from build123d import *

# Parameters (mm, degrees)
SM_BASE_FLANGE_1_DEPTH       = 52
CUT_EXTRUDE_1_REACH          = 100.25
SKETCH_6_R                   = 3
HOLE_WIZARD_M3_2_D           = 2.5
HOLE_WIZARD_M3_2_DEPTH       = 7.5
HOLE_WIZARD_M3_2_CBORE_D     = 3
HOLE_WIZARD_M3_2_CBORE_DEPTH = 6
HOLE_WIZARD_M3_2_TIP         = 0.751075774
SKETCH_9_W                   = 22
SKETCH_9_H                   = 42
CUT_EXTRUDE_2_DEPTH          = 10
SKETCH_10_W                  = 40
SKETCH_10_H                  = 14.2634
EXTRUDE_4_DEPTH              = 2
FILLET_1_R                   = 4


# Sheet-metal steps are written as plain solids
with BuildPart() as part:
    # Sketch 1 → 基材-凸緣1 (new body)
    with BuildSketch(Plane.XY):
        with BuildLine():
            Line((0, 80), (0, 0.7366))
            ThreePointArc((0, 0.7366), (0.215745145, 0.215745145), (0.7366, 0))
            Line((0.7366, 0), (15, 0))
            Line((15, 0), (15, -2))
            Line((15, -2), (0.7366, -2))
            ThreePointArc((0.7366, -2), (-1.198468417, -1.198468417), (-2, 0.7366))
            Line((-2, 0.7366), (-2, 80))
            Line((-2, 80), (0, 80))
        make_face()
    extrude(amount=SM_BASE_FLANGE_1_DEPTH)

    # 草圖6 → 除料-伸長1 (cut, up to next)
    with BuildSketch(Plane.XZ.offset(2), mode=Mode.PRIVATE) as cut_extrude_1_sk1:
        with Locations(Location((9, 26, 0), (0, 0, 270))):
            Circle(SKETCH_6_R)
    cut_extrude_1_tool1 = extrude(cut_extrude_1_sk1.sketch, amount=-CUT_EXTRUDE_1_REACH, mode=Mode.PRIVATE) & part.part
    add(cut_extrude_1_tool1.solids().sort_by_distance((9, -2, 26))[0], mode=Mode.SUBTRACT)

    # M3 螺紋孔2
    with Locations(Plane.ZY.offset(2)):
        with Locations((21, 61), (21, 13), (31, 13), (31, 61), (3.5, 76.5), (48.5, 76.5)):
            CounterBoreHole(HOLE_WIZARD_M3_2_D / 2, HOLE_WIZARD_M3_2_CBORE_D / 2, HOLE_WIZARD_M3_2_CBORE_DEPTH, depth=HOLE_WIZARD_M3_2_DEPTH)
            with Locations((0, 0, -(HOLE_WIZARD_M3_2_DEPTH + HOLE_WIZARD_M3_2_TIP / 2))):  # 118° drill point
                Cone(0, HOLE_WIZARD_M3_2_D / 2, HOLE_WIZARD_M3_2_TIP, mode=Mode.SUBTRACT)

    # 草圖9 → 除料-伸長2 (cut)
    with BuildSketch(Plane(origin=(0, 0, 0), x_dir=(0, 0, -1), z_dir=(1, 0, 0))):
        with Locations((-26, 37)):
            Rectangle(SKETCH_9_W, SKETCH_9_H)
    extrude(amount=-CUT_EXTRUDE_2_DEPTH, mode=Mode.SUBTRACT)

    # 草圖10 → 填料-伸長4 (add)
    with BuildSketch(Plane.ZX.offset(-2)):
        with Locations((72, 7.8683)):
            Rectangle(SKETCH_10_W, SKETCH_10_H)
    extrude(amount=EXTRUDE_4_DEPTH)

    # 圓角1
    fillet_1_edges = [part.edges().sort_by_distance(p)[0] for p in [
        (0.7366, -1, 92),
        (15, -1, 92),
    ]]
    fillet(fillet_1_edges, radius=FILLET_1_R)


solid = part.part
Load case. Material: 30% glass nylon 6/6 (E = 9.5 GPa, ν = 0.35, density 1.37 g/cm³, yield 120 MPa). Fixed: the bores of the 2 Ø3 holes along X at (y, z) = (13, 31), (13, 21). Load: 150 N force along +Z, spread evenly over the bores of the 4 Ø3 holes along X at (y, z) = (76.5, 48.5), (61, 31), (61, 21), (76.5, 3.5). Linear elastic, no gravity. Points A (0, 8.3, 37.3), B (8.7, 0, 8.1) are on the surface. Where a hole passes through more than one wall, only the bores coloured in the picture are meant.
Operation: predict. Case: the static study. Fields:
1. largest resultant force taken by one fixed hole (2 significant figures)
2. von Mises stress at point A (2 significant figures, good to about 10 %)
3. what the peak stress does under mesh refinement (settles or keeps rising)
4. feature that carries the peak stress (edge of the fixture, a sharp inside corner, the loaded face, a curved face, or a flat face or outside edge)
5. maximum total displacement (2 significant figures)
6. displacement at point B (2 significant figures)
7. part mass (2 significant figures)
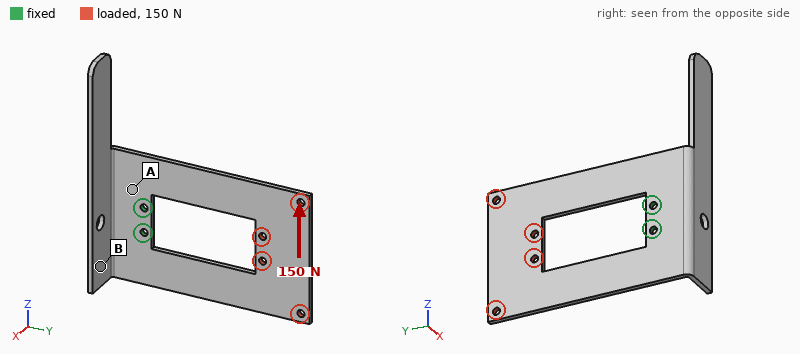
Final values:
620 N
18 MPa
keeps rising
edge of the fixture
1.0 mm
0.18 mm
13 g
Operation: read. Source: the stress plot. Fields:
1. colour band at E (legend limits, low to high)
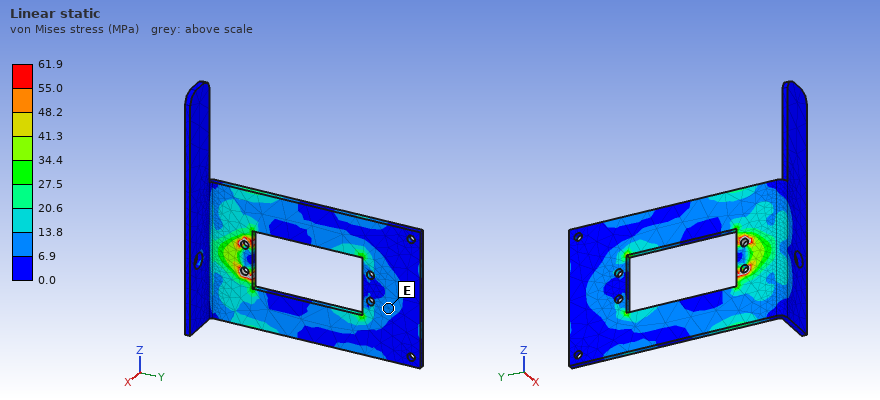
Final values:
6.9 to 13.8 MPa
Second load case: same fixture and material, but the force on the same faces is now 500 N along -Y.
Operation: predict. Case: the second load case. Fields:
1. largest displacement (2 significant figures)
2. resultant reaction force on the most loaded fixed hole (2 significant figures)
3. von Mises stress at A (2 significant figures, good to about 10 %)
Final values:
0.17 mm
290 N
16 MPa
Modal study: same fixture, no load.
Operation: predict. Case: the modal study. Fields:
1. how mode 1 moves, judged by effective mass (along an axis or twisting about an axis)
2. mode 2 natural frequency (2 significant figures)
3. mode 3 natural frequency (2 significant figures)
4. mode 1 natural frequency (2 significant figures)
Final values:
along X
370 Hz
380 Hz
130 Hz
